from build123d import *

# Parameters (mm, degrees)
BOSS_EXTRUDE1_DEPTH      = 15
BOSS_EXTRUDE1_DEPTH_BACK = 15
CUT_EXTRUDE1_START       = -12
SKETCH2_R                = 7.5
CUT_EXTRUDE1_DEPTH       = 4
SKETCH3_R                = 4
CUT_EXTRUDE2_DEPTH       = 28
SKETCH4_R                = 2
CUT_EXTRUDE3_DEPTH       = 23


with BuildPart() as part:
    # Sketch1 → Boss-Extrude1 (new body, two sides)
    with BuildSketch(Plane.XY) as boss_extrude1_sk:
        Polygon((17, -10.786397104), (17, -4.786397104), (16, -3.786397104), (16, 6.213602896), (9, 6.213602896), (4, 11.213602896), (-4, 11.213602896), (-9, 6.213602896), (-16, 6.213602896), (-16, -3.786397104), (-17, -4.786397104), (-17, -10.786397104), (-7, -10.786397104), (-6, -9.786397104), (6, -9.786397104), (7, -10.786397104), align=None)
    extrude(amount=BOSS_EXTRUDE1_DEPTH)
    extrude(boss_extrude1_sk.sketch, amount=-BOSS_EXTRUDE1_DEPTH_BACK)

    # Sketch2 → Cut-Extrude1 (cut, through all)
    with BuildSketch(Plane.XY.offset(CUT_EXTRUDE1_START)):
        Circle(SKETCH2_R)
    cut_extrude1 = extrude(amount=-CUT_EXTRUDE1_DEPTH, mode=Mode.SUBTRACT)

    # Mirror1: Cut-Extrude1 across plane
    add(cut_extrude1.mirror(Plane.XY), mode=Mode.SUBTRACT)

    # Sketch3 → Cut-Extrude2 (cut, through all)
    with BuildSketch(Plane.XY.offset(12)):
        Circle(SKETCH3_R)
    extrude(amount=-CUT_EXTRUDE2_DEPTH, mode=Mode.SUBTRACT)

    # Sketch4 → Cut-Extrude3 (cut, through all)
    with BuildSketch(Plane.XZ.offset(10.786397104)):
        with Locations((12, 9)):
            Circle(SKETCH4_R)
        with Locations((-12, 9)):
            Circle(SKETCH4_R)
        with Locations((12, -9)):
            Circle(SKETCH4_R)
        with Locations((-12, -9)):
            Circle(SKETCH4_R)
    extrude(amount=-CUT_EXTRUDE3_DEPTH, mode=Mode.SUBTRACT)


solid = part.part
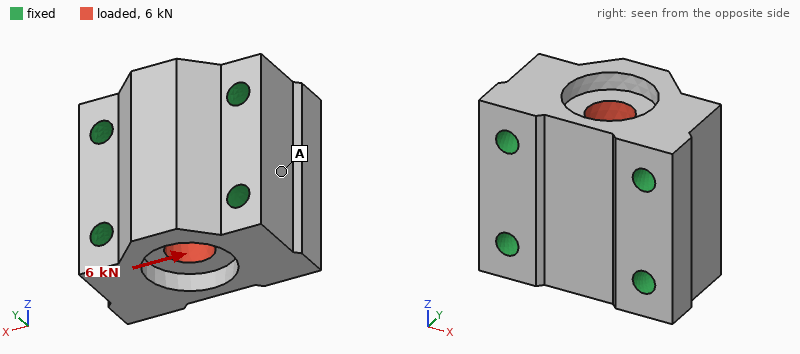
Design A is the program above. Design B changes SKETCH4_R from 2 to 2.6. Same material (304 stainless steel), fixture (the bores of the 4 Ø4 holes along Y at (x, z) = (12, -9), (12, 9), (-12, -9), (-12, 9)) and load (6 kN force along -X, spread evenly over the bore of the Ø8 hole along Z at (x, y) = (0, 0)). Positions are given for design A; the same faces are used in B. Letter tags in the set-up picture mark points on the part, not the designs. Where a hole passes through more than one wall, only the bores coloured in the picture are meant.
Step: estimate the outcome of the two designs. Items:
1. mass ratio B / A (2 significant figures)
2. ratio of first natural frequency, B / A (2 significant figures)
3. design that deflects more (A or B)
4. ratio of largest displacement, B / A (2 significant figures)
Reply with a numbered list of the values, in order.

1. 0.96
2. 1.1
3. A
4. 0.90
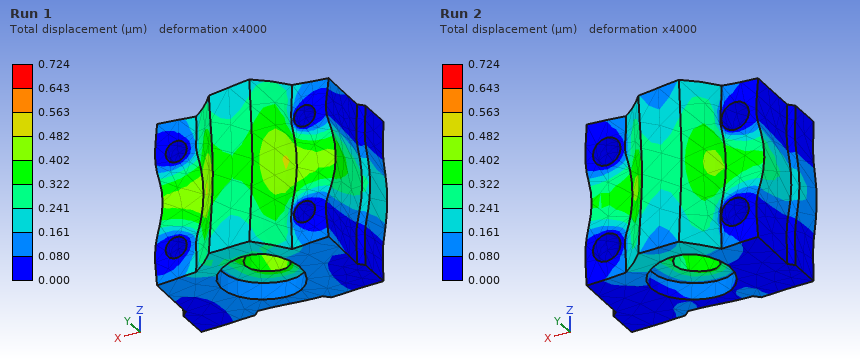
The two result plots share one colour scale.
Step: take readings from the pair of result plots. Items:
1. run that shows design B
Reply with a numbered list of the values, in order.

1. Run 2
